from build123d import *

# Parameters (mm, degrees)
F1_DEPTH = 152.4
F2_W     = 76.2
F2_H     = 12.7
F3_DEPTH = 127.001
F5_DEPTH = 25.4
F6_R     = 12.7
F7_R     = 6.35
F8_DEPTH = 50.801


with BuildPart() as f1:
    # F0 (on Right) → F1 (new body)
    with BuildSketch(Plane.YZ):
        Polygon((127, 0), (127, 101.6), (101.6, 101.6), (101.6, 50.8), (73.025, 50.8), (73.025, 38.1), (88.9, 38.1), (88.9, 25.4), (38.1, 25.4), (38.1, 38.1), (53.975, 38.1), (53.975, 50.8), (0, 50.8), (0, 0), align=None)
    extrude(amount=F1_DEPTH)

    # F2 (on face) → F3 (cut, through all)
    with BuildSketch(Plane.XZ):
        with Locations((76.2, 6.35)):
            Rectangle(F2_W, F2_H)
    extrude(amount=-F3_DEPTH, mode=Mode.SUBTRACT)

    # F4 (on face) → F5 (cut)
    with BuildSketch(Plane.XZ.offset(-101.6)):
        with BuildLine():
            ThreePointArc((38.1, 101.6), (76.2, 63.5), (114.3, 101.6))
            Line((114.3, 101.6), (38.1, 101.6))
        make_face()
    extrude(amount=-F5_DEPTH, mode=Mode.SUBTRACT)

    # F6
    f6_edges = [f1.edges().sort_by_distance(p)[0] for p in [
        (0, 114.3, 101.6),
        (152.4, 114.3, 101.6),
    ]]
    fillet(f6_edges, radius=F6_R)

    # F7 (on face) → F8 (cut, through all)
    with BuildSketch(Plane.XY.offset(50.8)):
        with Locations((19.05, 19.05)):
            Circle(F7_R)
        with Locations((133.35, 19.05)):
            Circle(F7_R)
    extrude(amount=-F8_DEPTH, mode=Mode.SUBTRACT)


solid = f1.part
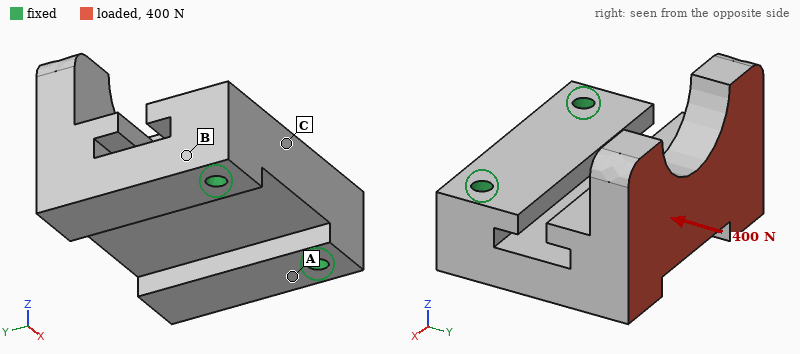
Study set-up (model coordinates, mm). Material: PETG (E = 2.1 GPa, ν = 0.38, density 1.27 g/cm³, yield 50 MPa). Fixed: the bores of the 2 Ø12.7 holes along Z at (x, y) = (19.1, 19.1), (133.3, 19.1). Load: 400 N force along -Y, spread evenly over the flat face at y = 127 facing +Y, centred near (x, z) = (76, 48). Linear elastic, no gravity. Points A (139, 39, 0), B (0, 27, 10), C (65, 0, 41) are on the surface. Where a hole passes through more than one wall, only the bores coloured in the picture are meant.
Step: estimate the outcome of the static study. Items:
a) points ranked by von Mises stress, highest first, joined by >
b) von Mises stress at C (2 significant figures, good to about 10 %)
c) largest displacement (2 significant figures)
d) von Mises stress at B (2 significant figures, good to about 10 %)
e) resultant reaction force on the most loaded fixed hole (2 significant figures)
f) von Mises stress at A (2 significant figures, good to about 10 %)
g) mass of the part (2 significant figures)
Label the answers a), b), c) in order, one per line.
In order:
a) A > B > C
b) 0.16 MPa
c) 0.38 mm
d) 0.44 MPa
e) 220 N
f) 1.1 MPa
g) 1.1 kg
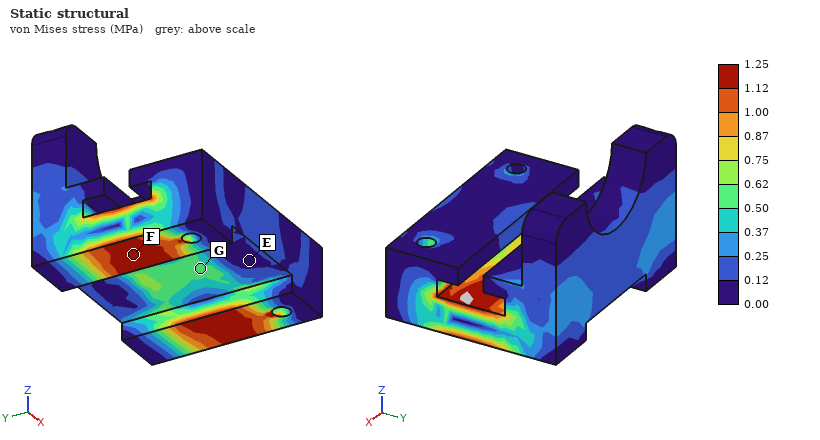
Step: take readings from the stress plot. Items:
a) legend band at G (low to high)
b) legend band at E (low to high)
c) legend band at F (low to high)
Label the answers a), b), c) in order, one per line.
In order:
a) 0.50 to 0.62 MPa
b) 0.00 to 0.12 MPa
c) 1.12 to 1.25 MPa
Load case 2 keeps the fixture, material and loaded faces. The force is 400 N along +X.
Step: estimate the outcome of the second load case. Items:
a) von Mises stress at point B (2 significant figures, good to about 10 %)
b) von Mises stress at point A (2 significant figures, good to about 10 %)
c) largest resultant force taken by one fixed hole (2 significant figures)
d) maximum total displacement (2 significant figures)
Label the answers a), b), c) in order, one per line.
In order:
a) 0.40 MPa
b) 0.80 MPa
c) 410 N
d) 98 µm
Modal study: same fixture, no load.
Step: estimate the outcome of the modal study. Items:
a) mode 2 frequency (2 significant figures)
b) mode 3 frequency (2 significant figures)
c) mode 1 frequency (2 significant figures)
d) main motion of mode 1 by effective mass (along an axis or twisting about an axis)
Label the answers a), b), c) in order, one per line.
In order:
a) 410 Hz
b) 730 Hz
c) 210 Hz
d) along Z
